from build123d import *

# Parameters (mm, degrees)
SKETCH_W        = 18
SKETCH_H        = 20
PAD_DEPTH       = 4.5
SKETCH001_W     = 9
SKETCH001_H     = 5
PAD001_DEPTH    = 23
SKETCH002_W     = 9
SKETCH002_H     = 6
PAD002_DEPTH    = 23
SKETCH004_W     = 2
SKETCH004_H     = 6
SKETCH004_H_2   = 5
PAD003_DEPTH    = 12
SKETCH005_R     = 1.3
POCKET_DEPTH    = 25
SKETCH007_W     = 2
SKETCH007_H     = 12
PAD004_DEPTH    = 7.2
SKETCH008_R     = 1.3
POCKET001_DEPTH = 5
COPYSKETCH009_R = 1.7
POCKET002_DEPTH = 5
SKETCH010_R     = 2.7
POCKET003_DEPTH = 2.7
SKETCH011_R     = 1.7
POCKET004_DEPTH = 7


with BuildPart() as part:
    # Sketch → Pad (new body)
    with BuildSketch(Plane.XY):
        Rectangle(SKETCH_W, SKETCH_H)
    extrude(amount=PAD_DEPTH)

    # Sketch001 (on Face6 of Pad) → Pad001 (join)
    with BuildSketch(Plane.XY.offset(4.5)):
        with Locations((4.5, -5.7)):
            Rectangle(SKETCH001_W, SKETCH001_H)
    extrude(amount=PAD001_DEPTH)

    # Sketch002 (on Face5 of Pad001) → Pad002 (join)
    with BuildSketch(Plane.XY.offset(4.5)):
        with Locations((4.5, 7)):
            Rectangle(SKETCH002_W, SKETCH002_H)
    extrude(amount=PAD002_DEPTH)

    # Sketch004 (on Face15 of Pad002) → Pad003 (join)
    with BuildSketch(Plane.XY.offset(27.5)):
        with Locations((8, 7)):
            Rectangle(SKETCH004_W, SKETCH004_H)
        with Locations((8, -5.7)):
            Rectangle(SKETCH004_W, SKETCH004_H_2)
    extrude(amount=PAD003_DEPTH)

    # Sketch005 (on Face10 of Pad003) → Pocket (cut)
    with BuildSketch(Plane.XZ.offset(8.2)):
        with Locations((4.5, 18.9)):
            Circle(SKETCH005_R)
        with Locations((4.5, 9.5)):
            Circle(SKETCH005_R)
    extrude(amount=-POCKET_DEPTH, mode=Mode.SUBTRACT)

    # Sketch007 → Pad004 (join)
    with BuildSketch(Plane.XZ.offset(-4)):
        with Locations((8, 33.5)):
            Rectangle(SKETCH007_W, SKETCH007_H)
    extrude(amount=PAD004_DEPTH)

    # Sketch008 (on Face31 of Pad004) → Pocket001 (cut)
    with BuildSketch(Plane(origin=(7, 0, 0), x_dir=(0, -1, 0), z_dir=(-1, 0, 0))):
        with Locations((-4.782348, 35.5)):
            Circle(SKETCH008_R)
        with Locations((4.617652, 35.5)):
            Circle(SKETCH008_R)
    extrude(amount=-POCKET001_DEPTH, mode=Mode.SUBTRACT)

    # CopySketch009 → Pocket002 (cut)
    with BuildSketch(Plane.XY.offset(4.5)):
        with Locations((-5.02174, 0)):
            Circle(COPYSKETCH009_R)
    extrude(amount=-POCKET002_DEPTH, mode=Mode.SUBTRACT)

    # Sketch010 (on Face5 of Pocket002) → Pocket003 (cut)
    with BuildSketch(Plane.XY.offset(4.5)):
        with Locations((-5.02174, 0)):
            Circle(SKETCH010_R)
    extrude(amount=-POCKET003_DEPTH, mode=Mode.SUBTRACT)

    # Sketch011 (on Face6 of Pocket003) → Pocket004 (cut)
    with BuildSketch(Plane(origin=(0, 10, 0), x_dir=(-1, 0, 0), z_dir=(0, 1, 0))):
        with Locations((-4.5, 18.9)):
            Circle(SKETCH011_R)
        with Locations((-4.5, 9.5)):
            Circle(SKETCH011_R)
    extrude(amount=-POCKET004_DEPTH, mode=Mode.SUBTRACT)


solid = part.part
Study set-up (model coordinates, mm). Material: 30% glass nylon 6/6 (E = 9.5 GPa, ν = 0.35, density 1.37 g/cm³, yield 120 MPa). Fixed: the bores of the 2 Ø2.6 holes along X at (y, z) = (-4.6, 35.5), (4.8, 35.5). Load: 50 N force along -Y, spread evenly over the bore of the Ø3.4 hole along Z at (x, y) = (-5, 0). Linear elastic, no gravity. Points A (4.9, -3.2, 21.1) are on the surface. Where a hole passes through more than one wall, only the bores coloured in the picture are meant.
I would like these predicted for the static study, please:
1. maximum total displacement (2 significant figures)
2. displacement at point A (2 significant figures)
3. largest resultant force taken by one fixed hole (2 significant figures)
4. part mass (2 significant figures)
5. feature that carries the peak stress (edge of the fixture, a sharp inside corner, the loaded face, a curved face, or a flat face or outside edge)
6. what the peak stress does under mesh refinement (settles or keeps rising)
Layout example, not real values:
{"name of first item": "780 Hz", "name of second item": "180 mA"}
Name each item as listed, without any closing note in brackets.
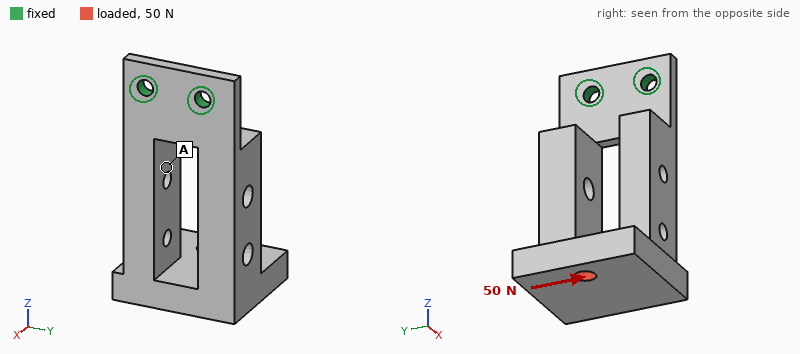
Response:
{"maximum total displacement": "0.48 mm", "displacement at point A": "0.10 mm", "largest resultant force taken by one fixed hole": "160 N", "part mass": "5.6 g", "feature that carries the peak stress": "edge of the fixture", "what the peak stress does under mesh refinement": "keeps rising"}
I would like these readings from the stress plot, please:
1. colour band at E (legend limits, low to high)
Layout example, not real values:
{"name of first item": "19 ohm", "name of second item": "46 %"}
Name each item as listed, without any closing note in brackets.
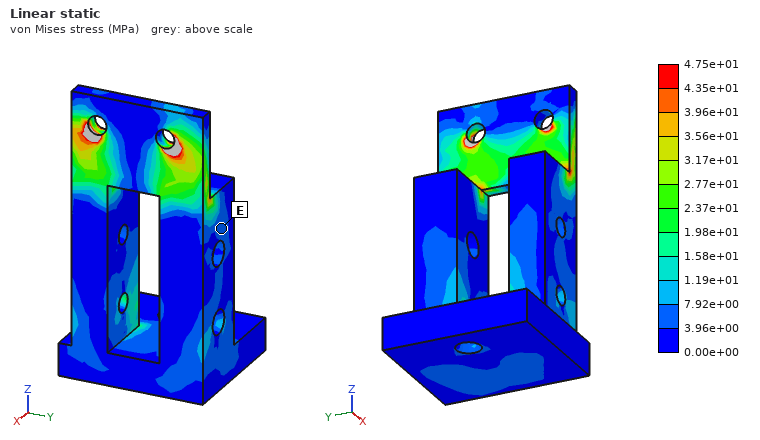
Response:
{"colour band at E": "3.96e+00 to 7.92e+00 MPa"}
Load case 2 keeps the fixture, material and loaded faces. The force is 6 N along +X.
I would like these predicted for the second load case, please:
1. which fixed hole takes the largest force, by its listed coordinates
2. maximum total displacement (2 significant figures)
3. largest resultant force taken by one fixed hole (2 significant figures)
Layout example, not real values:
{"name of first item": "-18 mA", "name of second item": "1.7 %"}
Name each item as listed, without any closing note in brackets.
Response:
{"which fixed hole takes the largest force, by its listed coordinates": "(4.8, 35.5)", "maximum total displacement": "0.54 mm", "largest resultant force taken by one fixed hole": "3.3 N"}
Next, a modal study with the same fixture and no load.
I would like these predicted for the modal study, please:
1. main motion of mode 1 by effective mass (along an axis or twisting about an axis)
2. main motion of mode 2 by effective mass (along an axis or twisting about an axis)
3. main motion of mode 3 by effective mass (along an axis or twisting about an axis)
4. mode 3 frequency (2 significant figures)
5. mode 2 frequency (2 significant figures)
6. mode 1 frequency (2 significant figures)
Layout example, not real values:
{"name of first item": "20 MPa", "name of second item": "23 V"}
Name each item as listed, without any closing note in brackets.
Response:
{"main motion of mode 1 by effective mass": "along X", "main motion of mode 2 by effective mass": "along Y", "main motion of mode 3 by effective mass": "along Y", "mode 3 frequency": "2000 Hz", "mode 2 frequency": "1300 Hz", "mode 1 frequency": "330 Hz"}
